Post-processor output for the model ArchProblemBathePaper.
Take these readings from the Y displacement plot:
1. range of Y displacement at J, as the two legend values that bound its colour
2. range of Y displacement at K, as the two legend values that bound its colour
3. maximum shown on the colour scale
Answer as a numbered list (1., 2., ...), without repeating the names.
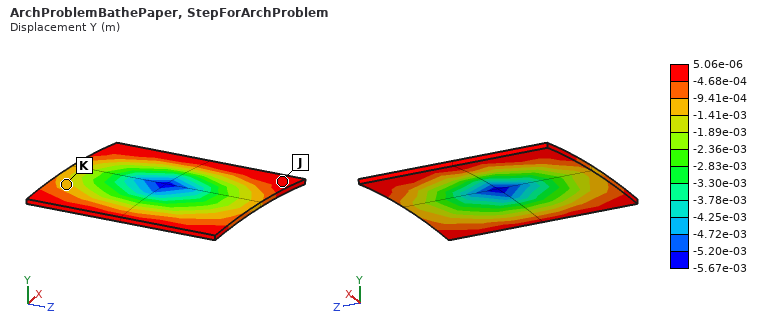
1. -4.68e-04 to 5.06e-06 m
2. -1.41e-03 to -9.41e-04 m
3. 5.06e-06 m
